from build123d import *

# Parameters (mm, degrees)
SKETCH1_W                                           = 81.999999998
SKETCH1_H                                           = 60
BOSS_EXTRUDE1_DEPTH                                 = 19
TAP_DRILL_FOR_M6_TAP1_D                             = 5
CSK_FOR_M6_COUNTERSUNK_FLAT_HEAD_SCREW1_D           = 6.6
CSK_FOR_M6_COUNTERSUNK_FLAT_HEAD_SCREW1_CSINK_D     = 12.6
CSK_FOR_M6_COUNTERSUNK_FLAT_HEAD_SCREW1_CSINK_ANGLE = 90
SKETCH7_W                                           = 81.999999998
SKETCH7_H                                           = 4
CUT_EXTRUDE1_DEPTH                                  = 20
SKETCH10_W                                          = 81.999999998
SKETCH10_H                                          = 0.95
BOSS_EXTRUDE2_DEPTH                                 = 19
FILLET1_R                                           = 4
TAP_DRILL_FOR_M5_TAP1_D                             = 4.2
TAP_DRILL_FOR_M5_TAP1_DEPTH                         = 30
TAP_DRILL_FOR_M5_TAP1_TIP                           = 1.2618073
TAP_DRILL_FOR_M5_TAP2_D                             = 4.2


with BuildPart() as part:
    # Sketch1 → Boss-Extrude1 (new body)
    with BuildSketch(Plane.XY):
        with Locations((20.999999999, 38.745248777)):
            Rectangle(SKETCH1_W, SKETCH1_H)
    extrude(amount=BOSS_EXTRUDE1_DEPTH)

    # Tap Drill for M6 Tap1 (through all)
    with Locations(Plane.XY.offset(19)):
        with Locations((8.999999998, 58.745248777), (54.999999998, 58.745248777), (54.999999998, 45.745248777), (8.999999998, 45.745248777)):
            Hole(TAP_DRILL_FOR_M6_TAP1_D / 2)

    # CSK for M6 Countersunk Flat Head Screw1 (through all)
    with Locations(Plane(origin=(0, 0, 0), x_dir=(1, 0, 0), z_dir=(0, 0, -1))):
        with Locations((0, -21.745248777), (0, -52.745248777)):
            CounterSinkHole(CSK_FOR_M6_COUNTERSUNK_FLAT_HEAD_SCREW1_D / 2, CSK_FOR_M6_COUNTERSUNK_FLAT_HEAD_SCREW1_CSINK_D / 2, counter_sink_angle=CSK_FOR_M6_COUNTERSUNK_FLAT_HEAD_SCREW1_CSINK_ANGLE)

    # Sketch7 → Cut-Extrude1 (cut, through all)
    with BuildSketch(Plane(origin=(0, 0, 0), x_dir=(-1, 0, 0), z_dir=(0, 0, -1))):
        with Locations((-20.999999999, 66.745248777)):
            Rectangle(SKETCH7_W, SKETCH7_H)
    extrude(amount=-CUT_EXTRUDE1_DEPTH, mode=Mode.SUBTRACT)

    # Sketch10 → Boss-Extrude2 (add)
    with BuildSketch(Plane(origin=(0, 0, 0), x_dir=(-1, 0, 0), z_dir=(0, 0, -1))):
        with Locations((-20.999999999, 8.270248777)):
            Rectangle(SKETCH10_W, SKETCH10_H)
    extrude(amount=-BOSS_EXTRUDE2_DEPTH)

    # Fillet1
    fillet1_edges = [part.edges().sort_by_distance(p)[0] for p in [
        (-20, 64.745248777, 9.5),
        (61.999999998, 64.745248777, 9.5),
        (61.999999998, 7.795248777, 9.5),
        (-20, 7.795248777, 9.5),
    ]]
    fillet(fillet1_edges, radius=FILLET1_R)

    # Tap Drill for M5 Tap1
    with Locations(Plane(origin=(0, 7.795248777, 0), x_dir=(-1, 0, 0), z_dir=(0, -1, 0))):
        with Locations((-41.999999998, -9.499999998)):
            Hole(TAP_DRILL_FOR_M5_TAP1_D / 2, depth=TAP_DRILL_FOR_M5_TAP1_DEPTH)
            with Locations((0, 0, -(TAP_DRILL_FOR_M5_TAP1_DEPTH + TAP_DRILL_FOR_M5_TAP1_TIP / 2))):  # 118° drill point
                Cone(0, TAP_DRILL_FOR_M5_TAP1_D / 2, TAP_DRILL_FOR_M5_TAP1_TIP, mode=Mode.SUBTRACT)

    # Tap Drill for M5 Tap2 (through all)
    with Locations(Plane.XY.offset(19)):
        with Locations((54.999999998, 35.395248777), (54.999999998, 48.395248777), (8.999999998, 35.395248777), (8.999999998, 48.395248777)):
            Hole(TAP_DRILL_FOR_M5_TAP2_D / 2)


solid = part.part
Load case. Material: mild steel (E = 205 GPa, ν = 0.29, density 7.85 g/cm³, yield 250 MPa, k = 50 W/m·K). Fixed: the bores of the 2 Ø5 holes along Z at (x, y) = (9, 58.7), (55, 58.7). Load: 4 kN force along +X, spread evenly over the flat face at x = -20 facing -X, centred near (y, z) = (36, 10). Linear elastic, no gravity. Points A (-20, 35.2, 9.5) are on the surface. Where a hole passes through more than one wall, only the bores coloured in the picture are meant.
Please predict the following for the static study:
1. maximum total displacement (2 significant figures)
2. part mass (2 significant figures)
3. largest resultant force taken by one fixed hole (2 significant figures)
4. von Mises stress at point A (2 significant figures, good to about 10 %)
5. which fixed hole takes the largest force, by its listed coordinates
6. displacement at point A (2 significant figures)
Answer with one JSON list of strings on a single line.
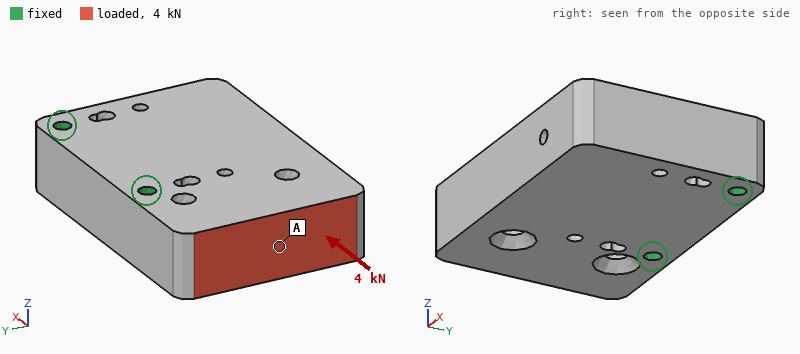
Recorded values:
["3.8 µm", "660 g", "3.2 kN", "3.7 MPa", "(9, 58.7)", "3.2 µm"]
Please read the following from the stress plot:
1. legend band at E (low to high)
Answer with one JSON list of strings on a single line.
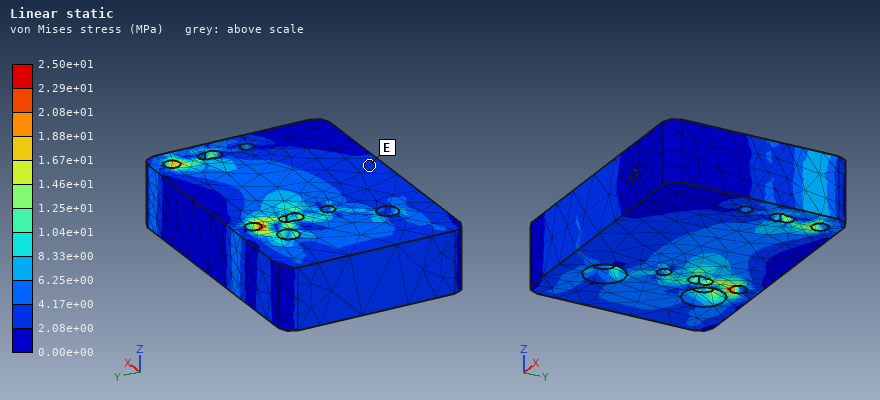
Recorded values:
["2.08e+00 to 4.17e+00 MPa"]
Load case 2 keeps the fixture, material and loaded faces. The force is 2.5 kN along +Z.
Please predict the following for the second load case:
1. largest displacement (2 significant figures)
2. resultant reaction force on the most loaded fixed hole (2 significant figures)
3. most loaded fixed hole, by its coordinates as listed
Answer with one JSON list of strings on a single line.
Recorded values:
["25 µm", "3.2 kN", "(9, 58.7)"]
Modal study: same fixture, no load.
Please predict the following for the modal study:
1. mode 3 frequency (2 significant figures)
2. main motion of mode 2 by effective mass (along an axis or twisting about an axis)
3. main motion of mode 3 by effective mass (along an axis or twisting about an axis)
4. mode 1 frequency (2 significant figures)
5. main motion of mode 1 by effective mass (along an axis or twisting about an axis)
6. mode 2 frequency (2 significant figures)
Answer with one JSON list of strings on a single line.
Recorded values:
["7800 Hz", "twisting about Y", "along X", "3700 Hz", "along Z", "6600 Hz"]
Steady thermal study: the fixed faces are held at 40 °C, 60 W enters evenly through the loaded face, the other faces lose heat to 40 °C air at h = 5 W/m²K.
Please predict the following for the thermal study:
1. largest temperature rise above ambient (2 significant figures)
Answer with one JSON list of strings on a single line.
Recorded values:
["63 K"]
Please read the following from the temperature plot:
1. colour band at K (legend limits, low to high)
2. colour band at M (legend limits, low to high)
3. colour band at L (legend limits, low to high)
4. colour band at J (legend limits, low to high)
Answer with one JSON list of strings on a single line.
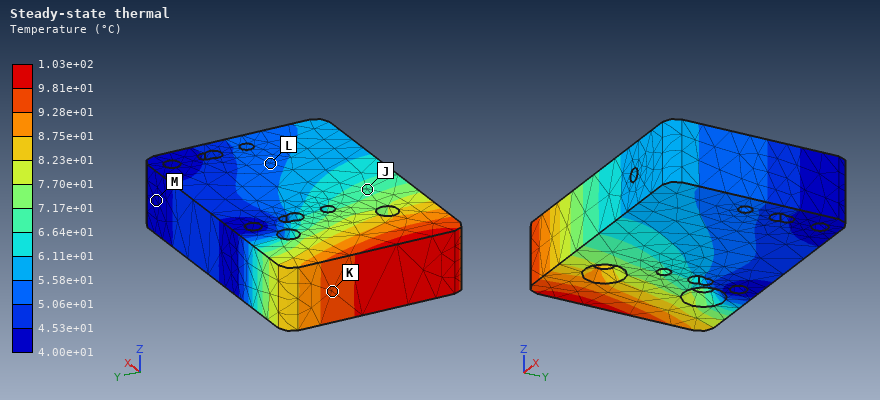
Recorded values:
["9.28e+01 to 9.81e+01 °C", "4.00e+01 to 4.53e+01 °C", "5.06e+01 to 5.58e+01 °C", "6.64e+01 to 7.17e+01 °C"]
